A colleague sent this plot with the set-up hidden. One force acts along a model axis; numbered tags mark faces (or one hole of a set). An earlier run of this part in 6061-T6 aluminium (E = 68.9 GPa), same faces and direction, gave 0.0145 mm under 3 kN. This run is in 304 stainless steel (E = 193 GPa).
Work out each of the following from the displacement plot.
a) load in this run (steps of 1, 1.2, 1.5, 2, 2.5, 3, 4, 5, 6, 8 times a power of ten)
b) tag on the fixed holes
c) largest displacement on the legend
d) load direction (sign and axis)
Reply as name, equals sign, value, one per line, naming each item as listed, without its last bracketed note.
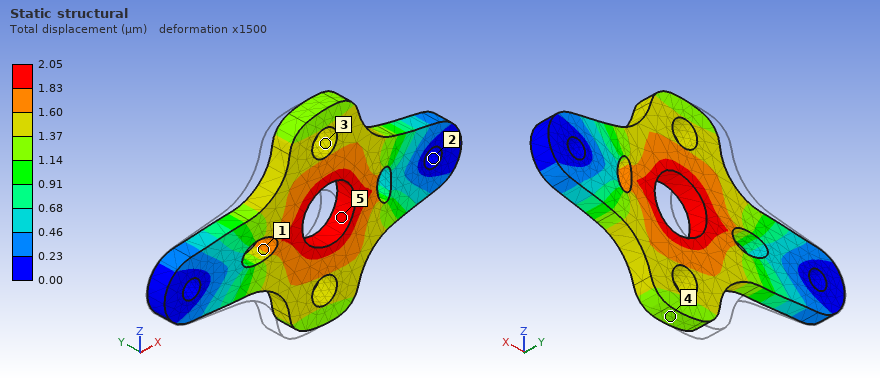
load in this run = 1.2 kN
tag on the fixed holes = 2
largest displacement on the legend = 2.05 µm
load direction = +X
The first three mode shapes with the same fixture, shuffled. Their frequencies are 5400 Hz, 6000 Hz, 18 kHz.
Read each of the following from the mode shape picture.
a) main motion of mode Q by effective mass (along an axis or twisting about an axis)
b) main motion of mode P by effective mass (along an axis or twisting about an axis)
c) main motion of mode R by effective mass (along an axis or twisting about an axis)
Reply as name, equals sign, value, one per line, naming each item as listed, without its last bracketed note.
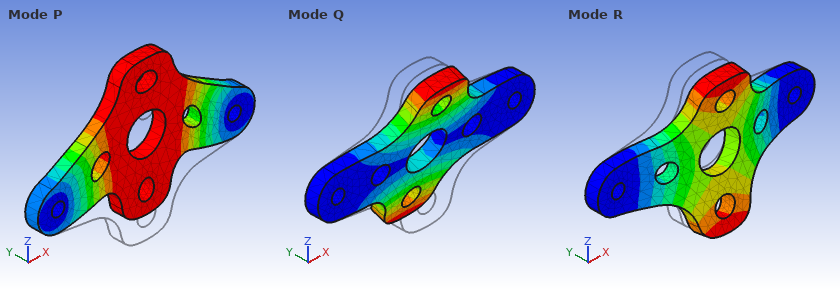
main motion of mode Q by effective mass = twisting about X
main motion of mode P by effective mass = along Z
main motion of mode R by effective mass = along Y
